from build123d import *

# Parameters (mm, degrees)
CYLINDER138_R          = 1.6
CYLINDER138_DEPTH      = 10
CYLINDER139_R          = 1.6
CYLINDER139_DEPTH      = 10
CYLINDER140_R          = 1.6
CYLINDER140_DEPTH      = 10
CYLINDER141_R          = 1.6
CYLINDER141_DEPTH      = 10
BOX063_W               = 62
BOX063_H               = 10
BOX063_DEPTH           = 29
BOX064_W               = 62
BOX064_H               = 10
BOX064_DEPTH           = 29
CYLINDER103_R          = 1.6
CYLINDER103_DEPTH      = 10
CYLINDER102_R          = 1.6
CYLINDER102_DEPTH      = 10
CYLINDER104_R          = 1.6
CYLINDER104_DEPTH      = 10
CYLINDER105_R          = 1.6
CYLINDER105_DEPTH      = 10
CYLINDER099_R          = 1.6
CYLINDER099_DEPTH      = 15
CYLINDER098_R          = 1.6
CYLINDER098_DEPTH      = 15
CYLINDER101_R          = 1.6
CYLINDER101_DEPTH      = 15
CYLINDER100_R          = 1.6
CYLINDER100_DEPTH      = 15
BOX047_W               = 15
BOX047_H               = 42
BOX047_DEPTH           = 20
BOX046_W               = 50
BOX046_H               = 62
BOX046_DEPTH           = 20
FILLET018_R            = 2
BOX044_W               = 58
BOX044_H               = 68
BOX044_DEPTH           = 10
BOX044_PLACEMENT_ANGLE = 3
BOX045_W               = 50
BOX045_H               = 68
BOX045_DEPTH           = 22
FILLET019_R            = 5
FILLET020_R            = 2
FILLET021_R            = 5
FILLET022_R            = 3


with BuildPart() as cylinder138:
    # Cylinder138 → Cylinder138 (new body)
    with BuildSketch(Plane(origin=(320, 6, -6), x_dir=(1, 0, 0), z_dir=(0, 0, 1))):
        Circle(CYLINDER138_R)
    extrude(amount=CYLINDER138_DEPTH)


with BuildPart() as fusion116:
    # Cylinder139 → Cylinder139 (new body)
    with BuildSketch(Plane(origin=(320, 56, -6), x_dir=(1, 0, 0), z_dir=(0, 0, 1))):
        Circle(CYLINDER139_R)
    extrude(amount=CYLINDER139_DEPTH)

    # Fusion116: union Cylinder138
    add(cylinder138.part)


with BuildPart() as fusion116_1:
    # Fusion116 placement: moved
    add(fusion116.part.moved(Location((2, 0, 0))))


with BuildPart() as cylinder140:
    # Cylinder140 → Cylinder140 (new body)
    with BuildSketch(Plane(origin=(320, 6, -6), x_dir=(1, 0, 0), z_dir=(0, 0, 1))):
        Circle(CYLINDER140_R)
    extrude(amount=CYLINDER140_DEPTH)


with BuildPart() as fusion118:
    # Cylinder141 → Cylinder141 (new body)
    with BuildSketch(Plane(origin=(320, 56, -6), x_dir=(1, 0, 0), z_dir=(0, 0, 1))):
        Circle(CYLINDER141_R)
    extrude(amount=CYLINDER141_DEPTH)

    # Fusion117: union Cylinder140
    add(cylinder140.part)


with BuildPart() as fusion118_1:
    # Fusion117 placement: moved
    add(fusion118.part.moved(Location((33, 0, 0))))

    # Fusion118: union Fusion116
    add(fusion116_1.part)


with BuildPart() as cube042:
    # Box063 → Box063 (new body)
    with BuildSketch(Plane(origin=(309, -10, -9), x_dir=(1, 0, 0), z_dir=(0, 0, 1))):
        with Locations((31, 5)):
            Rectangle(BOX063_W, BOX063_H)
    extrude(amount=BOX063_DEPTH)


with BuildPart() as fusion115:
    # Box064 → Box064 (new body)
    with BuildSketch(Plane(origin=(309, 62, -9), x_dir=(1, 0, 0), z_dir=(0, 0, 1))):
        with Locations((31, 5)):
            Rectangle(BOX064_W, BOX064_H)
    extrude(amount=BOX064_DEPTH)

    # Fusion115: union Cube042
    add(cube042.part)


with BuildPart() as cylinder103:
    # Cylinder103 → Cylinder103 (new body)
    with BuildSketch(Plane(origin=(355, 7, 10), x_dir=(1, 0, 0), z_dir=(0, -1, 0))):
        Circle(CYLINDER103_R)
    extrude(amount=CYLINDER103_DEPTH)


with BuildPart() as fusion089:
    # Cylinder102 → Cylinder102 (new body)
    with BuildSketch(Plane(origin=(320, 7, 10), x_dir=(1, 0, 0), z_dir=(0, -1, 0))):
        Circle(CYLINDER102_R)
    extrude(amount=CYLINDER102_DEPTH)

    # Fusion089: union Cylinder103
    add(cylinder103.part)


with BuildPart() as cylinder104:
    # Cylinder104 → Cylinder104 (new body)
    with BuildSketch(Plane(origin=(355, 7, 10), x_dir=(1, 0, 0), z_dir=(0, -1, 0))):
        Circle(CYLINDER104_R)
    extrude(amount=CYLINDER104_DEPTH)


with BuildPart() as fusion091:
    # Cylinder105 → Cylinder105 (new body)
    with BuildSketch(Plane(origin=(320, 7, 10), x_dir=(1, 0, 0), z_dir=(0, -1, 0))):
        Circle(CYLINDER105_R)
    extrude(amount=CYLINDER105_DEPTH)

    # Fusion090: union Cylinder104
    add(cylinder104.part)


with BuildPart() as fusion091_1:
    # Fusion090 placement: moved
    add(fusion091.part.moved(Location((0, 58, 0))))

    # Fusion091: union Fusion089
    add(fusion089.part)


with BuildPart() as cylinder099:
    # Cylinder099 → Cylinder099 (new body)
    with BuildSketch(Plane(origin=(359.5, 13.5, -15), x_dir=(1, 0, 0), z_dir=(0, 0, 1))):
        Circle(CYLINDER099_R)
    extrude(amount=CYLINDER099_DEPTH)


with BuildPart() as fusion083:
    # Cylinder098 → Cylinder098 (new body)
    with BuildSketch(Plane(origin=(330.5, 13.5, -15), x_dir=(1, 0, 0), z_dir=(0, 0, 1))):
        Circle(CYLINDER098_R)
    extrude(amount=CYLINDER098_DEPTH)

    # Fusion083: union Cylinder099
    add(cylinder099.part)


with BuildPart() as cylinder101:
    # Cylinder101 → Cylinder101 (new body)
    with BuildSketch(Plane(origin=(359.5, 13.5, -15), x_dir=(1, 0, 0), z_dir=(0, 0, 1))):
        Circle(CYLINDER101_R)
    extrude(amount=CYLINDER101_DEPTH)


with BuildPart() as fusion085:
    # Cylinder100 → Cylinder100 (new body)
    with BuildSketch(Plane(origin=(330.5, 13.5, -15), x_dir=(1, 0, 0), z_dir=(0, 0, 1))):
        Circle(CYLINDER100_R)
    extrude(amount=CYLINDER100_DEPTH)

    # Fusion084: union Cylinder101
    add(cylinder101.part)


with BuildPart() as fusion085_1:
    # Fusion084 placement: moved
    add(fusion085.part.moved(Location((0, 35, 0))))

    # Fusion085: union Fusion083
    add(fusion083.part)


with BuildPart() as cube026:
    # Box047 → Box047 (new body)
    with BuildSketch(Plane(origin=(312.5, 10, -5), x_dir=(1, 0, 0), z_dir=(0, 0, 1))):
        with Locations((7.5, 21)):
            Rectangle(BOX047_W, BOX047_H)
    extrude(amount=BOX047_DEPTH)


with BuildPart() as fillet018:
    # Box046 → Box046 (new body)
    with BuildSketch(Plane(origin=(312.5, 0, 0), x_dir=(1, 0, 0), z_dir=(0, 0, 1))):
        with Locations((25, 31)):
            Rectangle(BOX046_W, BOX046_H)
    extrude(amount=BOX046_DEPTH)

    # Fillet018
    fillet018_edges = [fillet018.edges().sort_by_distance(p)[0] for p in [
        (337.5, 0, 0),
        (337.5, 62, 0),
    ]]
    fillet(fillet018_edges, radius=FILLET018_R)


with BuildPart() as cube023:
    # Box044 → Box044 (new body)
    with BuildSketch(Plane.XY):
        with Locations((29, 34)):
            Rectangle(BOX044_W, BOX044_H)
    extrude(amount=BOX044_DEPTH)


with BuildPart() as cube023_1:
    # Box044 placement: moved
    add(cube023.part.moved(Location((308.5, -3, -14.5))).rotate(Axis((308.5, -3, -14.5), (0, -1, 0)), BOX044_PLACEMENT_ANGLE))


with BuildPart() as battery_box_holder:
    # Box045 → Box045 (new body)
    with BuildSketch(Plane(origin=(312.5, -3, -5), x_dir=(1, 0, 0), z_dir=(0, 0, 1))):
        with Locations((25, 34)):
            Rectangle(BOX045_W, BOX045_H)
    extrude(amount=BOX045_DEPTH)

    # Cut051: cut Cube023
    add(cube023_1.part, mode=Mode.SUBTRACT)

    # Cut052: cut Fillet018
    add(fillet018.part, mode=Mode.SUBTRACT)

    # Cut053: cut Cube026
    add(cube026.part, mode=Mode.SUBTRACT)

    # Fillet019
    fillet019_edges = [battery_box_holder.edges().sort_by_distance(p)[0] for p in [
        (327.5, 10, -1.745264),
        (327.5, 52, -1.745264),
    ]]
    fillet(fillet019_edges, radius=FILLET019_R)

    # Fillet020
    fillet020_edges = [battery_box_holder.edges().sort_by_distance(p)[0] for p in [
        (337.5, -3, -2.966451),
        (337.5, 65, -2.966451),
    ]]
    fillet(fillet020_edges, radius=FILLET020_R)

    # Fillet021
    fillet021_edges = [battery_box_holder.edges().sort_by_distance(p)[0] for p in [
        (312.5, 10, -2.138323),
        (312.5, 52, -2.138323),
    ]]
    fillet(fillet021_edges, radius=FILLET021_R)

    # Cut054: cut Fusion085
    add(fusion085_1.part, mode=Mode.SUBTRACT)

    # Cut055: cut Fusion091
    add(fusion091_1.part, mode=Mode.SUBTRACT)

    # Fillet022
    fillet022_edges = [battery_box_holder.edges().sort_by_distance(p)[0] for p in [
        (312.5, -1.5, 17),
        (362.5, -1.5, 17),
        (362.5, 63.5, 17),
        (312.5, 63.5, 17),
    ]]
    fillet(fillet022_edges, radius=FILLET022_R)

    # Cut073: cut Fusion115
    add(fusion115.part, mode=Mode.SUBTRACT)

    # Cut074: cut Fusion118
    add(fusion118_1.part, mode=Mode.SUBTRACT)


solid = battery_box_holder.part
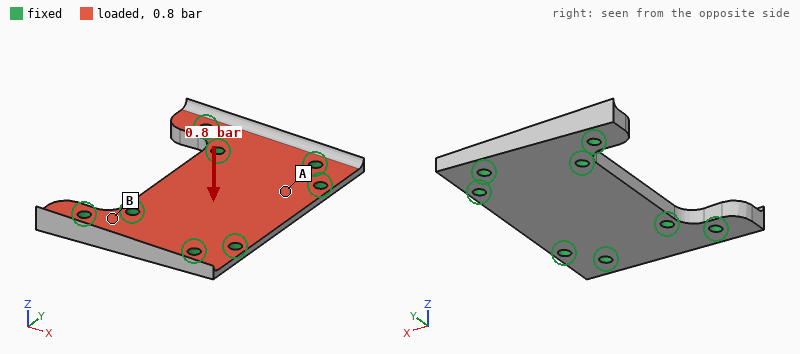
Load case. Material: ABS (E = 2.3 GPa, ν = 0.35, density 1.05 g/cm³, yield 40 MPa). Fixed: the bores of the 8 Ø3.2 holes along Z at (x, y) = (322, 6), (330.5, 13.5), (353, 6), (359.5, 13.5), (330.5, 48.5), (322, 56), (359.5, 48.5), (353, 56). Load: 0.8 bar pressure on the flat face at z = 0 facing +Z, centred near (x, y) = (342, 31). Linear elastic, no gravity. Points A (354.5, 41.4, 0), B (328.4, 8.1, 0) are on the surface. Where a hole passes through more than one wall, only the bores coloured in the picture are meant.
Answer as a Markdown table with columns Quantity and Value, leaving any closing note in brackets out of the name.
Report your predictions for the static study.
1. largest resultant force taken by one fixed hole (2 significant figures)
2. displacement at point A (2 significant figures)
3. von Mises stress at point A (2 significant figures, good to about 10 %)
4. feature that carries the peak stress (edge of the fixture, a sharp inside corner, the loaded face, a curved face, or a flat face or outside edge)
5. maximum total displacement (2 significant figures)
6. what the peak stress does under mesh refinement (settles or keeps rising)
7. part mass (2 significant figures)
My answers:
| Quantity | Value |
|---|---|
| largest resultant force taken by one fixed hole | 39 N |
| displacement at point A | 0.11 mm |
| von Mises stress at point A | 3.2 MPa |
| feature that carries the peak stress | edge of the fixture |
| maximum total displacement | 0.23 mm |
| what the peak stress does under mesh refinement | keeps rising |
| part mass | 7.0 g |
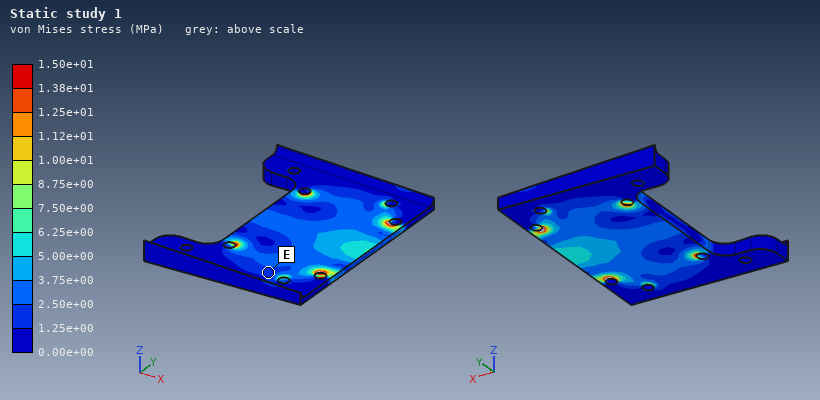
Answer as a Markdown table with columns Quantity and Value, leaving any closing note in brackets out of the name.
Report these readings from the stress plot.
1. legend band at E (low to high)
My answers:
| Quantity | Value |
|---|---|
| legend band at E | 1.25e+00 to 2.50e+00 MPa |
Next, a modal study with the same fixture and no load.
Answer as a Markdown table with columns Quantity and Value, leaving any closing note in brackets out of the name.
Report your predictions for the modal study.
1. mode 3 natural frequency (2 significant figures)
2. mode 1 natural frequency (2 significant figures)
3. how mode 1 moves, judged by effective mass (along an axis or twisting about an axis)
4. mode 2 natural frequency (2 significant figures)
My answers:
| Quantity | Value |
|---|---|
| mode 3 natural frequency | 5600 Hz |
| mode 1 natural frequency | 2500 Hz |
| how mode 1 moves, judged by effective mass | along Z |
| mode 2 natural frequency | 4000 Hz |
